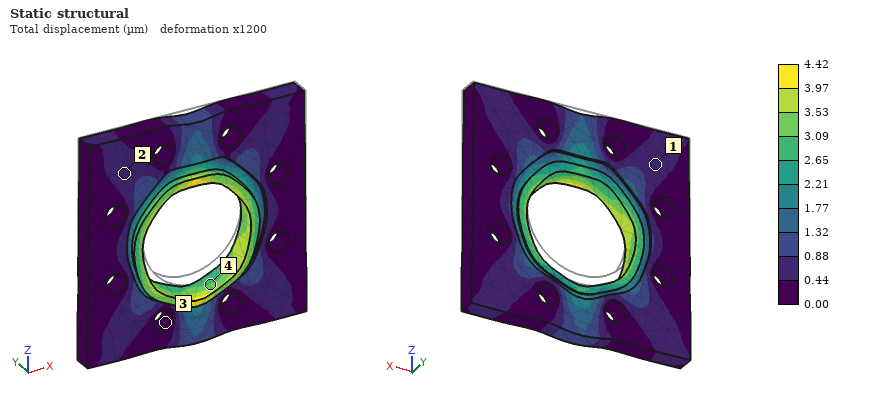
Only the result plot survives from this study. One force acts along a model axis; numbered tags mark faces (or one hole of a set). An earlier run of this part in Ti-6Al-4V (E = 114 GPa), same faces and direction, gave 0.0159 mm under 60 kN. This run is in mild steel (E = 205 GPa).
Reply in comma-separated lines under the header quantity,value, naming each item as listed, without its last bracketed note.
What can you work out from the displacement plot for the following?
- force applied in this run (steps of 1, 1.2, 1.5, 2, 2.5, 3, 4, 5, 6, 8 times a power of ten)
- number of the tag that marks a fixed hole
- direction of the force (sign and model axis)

quantity,value
force applied in this run,30 kN
number of the tag that marks a fixed hole,3
direction of the force,-Z
